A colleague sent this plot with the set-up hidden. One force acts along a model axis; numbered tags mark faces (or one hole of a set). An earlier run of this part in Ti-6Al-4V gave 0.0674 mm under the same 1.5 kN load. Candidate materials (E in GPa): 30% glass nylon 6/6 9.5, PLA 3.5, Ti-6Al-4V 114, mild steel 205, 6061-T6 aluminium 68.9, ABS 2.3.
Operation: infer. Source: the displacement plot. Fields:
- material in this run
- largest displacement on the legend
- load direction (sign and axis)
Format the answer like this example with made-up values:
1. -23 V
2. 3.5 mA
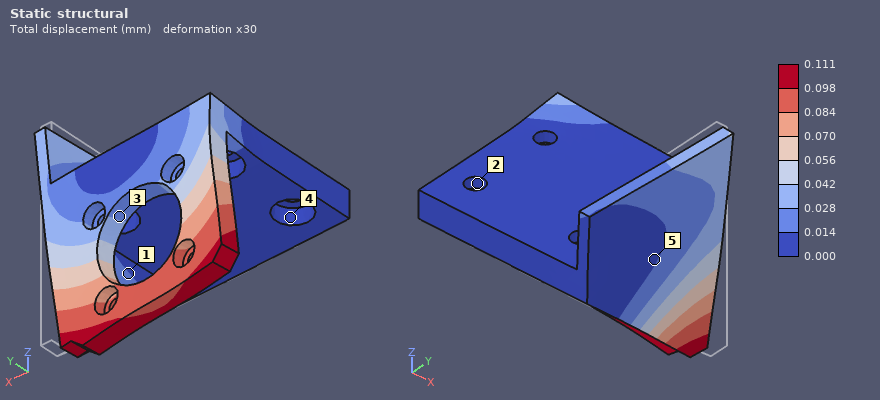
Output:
1. 6061-T6 aluminium
2. 0.111 mm
3. -X
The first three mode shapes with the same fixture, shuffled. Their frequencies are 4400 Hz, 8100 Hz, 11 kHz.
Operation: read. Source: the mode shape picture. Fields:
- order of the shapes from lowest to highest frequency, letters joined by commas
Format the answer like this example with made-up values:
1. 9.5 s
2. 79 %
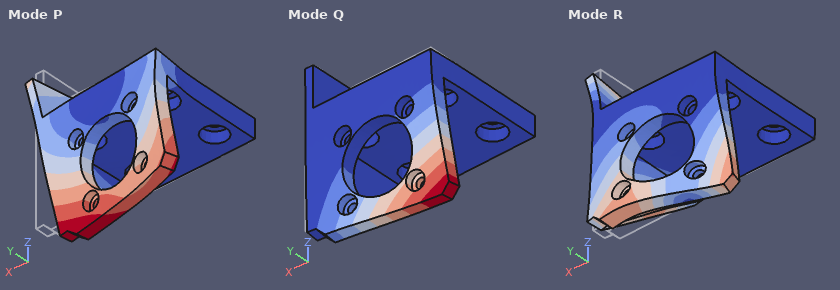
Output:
1. Q, P, R
